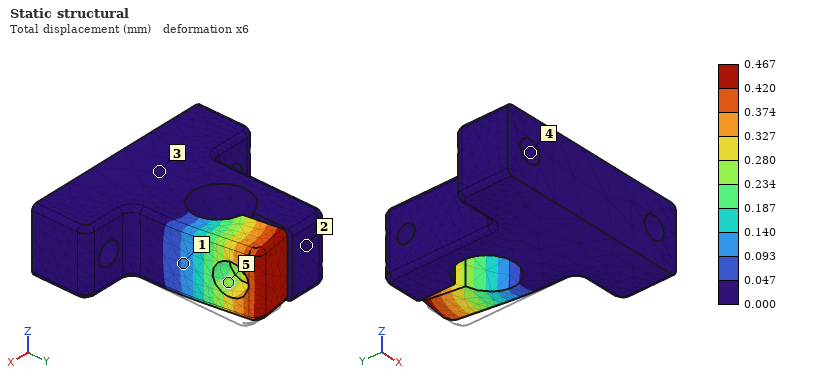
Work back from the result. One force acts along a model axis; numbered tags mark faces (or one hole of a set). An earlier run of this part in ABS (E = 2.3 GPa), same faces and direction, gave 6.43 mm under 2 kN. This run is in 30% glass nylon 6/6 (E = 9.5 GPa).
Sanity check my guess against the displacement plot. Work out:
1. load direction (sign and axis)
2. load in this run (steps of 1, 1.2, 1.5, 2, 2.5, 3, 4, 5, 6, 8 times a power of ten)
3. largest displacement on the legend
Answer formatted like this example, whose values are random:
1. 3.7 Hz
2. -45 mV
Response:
1. -X
2. 600 N
3. 0.467 mm
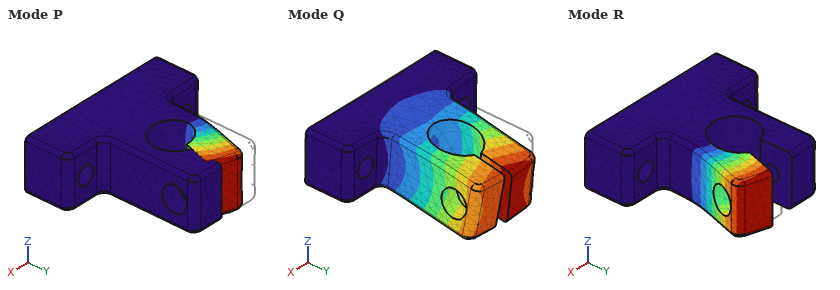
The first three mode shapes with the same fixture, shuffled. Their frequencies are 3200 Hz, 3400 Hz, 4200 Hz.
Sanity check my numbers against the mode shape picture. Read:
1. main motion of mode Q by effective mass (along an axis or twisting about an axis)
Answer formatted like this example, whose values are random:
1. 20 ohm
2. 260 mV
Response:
1. along Z
